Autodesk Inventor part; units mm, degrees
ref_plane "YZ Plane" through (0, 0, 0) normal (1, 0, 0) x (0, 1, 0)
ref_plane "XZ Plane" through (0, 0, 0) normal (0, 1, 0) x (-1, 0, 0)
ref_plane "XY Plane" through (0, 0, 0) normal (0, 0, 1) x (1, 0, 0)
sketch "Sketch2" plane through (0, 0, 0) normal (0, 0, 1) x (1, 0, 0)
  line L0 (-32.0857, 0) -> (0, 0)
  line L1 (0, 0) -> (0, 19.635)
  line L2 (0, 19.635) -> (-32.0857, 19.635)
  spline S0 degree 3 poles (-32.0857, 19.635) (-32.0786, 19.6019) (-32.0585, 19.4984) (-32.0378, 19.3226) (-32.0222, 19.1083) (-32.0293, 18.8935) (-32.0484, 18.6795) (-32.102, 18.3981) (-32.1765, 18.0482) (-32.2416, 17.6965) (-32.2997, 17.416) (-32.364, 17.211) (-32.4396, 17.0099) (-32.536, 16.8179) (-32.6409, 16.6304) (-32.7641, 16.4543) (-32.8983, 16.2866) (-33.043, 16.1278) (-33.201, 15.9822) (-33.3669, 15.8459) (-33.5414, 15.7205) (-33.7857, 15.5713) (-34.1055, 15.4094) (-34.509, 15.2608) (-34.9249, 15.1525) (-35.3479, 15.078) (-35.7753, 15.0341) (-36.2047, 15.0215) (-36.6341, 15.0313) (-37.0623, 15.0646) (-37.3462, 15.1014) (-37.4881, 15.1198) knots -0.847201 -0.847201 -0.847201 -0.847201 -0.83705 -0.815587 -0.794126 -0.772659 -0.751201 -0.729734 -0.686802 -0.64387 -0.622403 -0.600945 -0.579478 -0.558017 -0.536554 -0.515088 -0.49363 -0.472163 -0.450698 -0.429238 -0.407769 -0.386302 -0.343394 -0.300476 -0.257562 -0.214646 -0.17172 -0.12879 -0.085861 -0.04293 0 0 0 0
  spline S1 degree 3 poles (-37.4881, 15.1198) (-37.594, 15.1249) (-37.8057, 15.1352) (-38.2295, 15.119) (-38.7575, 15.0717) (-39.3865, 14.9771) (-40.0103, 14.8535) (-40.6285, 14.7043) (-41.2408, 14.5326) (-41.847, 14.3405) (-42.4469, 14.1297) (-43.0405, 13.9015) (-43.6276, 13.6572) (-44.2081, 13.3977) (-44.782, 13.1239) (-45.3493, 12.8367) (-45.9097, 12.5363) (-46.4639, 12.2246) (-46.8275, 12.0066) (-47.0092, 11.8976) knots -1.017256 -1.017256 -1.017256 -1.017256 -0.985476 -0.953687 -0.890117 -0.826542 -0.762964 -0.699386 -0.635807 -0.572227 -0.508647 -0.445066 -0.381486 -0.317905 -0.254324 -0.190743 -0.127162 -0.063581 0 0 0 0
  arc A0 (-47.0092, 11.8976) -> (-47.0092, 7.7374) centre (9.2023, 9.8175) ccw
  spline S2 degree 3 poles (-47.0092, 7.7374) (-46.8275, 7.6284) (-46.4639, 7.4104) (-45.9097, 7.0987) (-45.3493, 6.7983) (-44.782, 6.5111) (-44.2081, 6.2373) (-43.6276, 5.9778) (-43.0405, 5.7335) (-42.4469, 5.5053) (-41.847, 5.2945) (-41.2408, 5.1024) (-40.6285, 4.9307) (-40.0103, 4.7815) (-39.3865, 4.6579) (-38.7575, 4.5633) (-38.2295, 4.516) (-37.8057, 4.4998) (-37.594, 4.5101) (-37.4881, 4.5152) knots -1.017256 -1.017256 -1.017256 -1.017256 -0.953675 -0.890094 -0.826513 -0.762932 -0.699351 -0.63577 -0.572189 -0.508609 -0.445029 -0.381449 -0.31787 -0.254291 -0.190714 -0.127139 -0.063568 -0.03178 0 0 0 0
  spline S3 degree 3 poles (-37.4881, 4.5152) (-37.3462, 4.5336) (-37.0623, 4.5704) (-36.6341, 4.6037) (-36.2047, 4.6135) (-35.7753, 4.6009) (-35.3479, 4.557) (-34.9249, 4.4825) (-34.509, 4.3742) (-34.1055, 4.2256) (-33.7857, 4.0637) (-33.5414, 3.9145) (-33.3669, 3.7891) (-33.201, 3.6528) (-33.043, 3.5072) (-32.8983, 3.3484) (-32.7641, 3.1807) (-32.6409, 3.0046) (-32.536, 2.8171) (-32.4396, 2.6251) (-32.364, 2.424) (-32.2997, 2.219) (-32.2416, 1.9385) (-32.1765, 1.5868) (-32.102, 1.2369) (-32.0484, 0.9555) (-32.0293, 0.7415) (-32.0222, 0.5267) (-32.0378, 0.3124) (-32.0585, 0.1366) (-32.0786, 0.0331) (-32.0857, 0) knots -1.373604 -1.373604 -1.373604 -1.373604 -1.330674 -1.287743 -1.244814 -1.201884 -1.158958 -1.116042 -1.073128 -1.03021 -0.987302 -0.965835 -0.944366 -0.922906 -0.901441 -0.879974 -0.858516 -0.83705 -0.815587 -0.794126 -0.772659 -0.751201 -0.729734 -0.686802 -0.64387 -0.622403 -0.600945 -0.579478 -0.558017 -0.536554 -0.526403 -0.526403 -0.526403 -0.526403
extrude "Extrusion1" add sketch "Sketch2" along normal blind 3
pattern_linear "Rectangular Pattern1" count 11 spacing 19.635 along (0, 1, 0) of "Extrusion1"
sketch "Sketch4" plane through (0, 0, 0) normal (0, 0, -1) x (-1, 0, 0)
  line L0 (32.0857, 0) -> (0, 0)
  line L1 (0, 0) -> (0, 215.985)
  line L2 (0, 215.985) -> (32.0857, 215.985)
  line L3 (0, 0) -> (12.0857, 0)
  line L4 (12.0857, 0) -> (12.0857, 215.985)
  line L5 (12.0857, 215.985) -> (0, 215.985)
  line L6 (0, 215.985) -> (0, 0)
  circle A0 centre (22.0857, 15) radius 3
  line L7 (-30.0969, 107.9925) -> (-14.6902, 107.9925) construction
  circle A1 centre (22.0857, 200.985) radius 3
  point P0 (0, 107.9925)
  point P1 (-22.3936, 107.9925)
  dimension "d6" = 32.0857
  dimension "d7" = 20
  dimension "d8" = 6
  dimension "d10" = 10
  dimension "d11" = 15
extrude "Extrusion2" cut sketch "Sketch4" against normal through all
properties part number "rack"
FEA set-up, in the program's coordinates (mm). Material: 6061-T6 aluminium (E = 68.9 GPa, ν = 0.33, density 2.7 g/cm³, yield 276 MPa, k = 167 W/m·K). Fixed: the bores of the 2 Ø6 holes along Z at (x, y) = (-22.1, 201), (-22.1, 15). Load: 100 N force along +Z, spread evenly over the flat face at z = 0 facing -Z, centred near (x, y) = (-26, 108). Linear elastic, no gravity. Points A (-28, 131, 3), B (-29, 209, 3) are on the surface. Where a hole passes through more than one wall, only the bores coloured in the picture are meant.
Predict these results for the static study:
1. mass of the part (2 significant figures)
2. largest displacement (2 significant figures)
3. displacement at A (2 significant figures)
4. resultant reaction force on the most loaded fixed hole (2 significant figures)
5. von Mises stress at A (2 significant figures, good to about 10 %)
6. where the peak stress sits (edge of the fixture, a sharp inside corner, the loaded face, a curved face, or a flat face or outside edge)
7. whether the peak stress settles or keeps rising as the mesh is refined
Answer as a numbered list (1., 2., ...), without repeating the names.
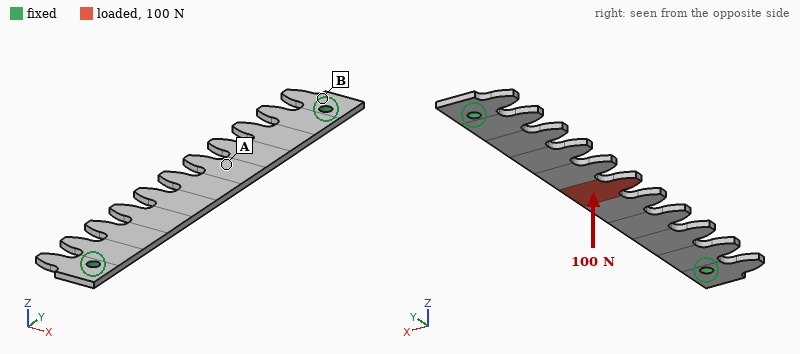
1. 47 g
2. 1.1 mm
3. 0.81 mm
4. 50 N
5. 33 MPa
6. edge of the fixture
7. keeps rising
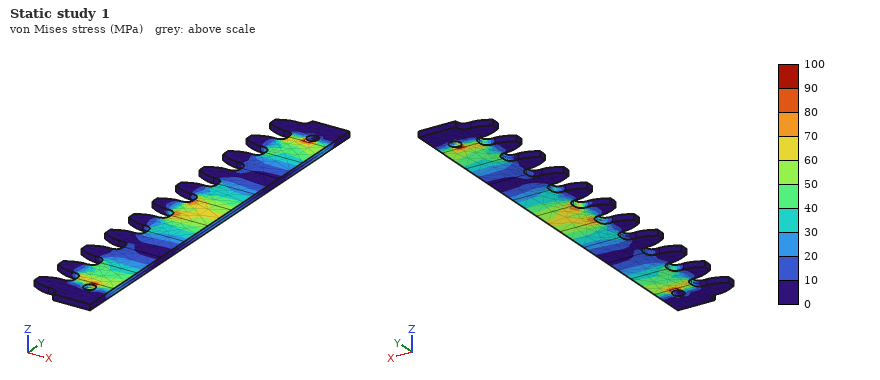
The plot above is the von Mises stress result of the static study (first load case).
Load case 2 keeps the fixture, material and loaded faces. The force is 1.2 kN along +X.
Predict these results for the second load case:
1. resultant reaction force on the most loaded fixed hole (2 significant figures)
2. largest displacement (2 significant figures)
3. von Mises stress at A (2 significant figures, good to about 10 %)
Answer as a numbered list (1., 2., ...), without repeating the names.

1. 600 N
2. 0.61 mm
3. 52 MPa
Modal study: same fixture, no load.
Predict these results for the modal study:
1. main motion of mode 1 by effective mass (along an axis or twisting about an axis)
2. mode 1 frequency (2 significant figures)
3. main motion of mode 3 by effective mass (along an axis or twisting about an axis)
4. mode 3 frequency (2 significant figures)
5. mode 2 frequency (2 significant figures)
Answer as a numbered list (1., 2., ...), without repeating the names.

1. along Z
2. 410 Hz
3. twisting about Y
4. 1400 Hz
5. 1100 Hz
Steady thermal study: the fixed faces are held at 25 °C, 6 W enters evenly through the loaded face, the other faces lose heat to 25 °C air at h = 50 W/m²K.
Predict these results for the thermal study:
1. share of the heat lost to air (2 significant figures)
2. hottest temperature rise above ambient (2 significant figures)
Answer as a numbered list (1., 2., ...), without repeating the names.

1. 59 %
2. 17 K
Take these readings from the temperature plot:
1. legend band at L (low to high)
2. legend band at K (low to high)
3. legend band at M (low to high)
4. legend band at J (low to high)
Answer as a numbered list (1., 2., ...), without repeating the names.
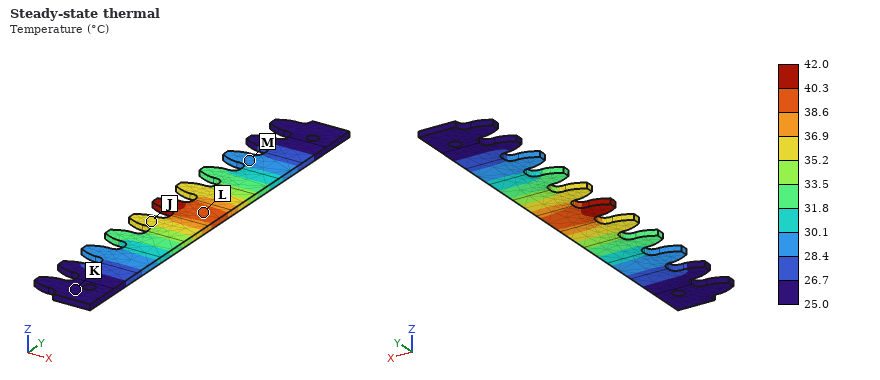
1. 38.6 to 40.3 °C
2. 25.0 to 26.7 °C
3. 28.4 to 30.1 °C
4. 35.2 to 36.9 °C
